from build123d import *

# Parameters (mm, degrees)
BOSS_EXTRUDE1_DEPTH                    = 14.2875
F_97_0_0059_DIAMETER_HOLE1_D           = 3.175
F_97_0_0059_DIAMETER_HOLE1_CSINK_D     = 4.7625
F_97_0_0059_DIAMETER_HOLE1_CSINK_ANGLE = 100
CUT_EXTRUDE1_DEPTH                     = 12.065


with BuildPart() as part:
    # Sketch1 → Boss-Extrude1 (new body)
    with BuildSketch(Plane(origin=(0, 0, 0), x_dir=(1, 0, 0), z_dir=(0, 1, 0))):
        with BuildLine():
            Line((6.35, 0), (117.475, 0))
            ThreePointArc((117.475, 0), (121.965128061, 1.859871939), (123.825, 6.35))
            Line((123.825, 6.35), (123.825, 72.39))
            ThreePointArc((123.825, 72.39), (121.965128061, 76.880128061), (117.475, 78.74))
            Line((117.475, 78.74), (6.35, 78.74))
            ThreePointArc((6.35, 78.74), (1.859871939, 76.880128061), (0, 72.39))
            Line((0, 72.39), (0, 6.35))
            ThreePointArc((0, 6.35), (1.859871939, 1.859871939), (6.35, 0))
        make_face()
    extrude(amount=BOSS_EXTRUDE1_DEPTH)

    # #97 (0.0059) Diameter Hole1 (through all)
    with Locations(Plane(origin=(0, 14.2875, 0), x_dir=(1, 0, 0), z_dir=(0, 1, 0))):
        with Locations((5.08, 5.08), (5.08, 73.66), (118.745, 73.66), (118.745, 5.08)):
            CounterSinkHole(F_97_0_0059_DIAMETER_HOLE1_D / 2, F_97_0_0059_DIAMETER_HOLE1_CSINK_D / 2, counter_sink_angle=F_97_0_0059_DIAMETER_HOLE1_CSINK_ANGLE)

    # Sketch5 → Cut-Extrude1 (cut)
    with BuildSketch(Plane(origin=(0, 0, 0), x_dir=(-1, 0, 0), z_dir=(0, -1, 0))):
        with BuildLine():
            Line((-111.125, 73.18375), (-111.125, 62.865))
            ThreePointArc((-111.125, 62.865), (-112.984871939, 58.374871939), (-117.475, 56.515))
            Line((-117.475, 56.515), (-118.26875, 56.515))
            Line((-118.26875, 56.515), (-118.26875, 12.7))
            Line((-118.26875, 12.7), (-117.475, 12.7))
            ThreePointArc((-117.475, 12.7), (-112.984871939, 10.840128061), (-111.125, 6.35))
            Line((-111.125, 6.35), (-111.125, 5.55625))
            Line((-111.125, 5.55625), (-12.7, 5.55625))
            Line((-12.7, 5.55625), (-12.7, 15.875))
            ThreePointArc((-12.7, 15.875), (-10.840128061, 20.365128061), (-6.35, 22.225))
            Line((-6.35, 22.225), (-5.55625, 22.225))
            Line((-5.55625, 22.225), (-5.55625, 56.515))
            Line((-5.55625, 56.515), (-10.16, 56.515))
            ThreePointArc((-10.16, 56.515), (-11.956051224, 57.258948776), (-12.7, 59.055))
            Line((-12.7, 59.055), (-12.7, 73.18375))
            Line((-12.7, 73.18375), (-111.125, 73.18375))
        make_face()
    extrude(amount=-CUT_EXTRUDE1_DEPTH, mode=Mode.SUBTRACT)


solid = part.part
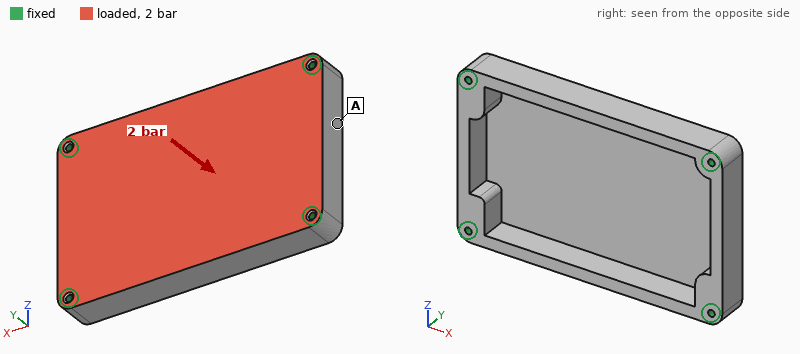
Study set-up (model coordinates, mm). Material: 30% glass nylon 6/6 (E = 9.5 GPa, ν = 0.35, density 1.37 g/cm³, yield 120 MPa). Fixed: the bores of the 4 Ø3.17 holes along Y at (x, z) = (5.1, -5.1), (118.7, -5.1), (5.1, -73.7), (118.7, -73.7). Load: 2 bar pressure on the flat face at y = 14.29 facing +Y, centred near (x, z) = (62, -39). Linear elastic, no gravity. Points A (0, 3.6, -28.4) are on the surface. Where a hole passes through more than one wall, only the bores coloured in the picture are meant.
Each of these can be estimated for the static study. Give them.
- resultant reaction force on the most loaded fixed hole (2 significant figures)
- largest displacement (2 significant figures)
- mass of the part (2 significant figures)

560 N
1.7 mm
70 g
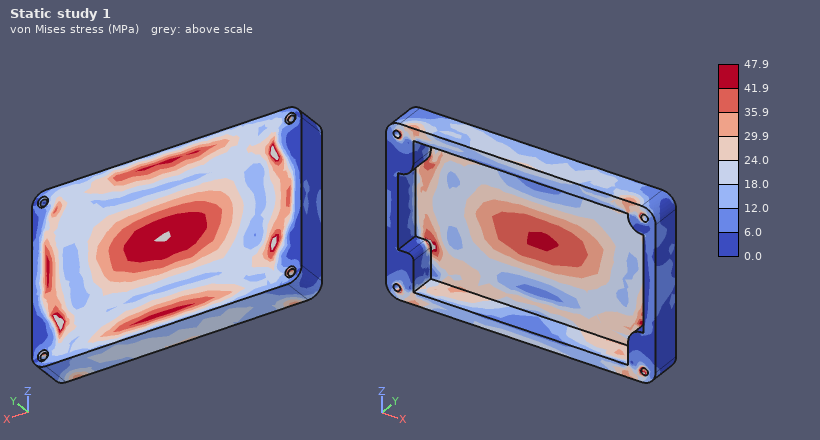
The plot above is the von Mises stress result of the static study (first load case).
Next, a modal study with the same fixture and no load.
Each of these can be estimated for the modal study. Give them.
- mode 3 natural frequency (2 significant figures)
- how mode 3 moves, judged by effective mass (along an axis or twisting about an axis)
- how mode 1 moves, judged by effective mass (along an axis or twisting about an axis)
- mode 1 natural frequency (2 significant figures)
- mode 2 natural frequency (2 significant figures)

2400 Hz
twisting about X
along Y
1200 Hz
2200 Hz
